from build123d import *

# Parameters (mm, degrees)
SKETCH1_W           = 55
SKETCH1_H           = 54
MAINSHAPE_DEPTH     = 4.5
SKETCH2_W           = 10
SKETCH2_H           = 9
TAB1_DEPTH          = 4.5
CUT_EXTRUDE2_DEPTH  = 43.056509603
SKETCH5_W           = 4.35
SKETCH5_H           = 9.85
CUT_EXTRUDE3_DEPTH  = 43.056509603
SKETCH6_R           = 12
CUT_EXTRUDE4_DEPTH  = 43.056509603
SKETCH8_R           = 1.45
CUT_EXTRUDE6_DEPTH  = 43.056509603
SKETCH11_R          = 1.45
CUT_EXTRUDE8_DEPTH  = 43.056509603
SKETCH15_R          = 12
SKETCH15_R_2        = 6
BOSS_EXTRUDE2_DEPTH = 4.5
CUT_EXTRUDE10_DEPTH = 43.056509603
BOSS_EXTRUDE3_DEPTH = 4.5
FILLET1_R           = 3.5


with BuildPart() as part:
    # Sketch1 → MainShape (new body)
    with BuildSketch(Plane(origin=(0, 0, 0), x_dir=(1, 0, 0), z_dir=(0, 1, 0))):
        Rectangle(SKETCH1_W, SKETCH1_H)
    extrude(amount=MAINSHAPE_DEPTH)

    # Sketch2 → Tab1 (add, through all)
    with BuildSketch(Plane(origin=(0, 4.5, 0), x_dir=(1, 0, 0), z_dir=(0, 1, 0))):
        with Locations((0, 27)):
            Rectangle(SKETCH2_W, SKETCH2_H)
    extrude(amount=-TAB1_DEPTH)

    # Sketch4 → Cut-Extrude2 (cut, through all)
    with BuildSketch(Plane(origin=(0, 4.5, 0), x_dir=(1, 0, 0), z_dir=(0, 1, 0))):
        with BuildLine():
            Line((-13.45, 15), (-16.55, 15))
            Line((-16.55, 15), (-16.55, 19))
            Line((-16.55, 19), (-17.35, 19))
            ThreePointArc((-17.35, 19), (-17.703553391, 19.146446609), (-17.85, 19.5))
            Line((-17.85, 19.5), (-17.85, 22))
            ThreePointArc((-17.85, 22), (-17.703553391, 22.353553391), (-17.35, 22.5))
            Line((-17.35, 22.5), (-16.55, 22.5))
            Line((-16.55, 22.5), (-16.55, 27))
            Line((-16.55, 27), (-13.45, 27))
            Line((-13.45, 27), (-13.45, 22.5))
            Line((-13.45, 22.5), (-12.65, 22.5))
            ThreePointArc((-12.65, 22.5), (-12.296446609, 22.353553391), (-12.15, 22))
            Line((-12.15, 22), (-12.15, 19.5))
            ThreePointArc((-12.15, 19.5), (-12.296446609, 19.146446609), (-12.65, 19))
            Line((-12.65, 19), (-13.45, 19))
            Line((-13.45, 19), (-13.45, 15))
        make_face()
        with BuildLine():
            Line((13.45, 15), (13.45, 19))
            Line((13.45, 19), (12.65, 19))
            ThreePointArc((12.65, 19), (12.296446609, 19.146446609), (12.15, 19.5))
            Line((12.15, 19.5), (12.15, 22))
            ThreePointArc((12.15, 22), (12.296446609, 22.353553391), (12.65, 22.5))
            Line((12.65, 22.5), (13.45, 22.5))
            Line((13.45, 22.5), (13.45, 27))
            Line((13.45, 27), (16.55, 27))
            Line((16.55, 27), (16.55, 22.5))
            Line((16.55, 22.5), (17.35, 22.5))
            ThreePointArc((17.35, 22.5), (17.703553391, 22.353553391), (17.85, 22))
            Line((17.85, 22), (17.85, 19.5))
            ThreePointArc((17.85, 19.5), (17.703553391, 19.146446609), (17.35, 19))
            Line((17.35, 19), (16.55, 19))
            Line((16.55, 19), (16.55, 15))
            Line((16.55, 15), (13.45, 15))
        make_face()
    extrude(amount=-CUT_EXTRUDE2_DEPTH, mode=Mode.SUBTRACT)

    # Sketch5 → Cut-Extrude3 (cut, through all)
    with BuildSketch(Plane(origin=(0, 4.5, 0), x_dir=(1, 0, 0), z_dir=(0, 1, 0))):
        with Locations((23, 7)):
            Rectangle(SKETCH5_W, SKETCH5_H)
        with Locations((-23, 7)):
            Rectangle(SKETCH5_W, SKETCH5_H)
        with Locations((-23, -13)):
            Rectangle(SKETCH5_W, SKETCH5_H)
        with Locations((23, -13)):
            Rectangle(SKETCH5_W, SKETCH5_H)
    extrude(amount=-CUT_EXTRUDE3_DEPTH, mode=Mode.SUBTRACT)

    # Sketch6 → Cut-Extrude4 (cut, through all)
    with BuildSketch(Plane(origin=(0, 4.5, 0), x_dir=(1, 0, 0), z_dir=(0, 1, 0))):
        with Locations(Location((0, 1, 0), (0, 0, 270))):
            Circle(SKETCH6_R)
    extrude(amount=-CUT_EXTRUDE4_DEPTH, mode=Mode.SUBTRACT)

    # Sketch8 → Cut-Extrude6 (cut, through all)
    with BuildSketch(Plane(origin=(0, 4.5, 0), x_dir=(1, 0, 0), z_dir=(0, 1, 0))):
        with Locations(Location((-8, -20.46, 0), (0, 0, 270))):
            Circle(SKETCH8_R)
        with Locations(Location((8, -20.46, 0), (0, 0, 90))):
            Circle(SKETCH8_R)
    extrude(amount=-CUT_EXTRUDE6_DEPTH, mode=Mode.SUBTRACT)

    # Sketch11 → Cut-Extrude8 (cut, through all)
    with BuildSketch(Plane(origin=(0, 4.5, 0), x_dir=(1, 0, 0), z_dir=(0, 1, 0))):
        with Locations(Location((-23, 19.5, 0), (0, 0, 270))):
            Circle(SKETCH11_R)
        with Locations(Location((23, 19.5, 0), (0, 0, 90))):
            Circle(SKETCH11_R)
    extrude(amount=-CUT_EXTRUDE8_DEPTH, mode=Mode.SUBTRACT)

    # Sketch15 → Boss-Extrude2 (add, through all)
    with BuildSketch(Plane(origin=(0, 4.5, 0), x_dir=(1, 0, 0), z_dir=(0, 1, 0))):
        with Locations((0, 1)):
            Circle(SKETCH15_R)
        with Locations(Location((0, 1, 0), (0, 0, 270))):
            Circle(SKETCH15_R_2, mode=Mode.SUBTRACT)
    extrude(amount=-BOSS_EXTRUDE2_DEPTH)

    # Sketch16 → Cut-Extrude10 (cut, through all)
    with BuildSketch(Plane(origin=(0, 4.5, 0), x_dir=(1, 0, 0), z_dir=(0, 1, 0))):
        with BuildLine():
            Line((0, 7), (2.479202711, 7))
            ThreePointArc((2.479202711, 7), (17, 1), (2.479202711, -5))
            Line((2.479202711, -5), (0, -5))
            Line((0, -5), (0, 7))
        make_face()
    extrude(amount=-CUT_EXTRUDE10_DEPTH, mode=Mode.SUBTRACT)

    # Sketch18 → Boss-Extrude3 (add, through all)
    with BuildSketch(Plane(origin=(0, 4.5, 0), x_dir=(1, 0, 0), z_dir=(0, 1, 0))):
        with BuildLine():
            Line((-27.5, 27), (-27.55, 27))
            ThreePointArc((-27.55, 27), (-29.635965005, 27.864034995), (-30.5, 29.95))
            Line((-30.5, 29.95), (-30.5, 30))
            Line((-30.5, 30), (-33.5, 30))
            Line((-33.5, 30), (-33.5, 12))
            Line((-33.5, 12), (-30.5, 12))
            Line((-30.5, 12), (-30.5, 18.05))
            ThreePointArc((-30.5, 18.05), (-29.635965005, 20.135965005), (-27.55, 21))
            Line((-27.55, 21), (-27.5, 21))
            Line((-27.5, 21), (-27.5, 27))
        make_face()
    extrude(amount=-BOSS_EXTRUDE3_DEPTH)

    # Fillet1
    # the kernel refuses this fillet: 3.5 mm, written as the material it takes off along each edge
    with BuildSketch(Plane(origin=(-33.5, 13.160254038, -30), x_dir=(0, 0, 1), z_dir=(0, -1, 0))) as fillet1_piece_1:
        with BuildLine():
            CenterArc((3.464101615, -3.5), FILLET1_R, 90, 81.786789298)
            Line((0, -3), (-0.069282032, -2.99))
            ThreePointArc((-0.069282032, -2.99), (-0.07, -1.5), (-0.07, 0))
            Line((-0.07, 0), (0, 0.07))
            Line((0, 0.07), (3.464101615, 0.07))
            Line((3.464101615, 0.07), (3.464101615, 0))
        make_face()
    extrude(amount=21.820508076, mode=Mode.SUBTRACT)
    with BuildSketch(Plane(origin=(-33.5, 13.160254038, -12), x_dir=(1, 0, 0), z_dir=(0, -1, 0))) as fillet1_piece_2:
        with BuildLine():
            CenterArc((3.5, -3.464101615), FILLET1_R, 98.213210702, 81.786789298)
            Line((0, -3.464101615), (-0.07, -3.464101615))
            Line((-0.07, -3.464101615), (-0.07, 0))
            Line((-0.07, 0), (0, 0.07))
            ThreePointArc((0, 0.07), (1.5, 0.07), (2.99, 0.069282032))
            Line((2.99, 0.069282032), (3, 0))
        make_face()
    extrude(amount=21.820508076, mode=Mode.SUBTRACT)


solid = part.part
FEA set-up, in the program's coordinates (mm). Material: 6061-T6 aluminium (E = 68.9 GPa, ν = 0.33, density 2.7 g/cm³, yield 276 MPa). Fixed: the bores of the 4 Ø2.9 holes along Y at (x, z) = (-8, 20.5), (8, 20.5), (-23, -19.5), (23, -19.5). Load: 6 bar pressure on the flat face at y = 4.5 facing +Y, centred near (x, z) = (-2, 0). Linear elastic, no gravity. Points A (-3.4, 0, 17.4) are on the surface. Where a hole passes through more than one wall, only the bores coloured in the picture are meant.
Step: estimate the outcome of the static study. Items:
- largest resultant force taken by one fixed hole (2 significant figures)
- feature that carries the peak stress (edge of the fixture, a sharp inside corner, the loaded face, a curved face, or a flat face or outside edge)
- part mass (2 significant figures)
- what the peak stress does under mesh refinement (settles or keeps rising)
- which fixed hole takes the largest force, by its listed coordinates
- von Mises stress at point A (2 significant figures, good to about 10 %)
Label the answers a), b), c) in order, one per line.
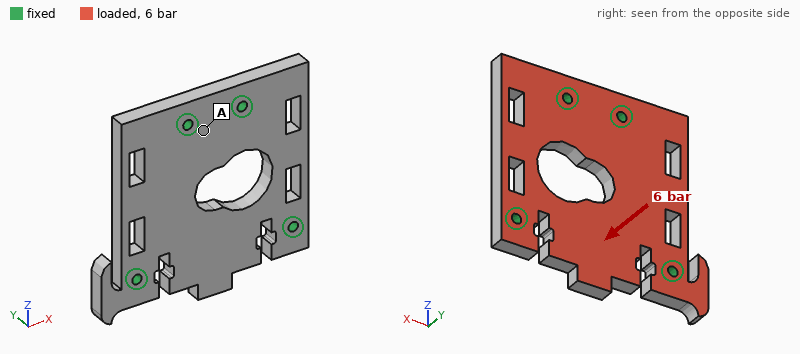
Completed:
a) 440 N
b) edge of the fixture
c) 30 g
d) keeps rising
e) (-23, -19.5)
f) 12 MPa
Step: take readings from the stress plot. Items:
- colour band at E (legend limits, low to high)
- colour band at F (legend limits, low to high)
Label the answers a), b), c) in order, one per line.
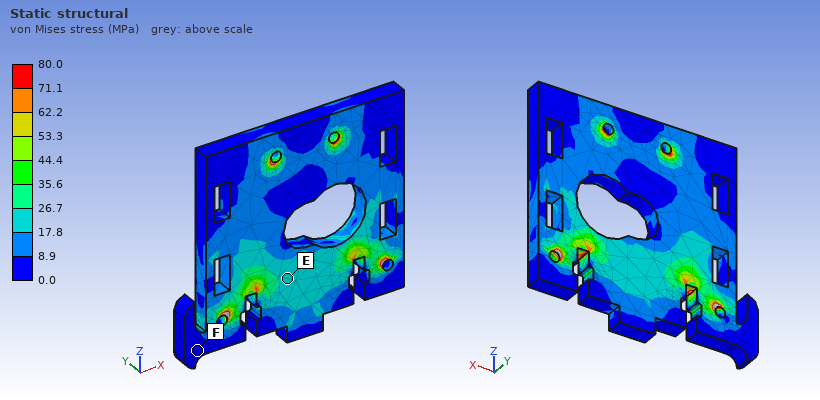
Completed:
a) 17.8 to 26.7 MPa
b) 0.0 to 8.9 MPa
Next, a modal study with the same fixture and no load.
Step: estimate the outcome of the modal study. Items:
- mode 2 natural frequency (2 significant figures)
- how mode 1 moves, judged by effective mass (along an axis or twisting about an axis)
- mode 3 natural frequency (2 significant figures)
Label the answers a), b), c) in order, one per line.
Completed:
a) 9100 Hz
b) along Y
c) 9200 Hz
